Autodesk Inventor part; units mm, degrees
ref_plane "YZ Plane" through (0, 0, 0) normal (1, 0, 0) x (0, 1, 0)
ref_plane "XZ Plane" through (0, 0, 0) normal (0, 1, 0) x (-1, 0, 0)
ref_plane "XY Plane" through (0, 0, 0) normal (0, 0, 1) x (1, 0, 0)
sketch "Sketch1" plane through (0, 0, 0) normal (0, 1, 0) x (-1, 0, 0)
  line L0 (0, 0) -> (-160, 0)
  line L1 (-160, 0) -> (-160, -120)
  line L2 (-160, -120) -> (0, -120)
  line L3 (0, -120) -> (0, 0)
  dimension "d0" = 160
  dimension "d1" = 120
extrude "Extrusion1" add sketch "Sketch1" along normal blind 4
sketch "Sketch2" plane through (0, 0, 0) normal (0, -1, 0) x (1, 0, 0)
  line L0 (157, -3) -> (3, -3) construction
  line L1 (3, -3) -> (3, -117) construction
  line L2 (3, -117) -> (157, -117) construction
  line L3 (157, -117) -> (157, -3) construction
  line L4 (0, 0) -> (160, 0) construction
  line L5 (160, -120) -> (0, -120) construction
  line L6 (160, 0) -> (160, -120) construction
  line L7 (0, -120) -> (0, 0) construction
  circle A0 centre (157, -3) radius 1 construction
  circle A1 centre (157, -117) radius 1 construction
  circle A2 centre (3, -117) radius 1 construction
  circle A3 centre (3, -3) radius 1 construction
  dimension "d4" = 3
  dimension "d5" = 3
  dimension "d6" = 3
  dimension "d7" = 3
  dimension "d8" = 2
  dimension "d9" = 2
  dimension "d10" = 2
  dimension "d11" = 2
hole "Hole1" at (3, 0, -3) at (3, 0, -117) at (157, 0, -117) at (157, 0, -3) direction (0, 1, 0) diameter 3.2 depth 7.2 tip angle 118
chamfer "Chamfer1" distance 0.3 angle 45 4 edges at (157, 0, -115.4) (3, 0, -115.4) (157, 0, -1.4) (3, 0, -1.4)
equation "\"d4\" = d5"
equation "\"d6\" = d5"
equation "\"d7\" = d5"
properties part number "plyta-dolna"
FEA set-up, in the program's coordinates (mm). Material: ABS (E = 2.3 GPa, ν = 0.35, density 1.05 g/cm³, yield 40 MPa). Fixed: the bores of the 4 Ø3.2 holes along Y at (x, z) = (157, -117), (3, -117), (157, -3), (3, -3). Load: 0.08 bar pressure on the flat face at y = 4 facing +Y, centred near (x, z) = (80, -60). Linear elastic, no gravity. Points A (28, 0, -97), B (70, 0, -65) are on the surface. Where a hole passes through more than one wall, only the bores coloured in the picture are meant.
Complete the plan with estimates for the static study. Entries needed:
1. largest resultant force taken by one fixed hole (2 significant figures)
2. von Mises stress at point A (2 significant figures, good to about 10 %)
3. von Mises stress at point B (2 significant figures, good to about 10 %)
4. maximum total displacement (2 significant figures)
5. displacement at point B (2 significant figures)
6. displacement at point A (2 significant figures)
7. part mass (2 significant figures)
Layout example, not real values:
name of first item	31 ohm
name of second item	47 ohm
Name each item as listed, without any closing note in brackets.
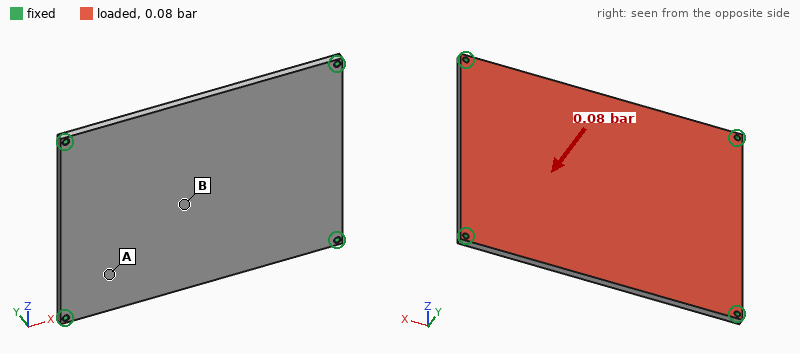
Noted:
largest resultant force taken by one fixed hole	38 N
von Mises stress at point A	1.8 MPa
von Mises stress at point B	4.0 MPa
maximum total displacement	2.3 mm
displacement at point B	2.2 mm
displacement at point A	1.0 mm
part mass	81 g
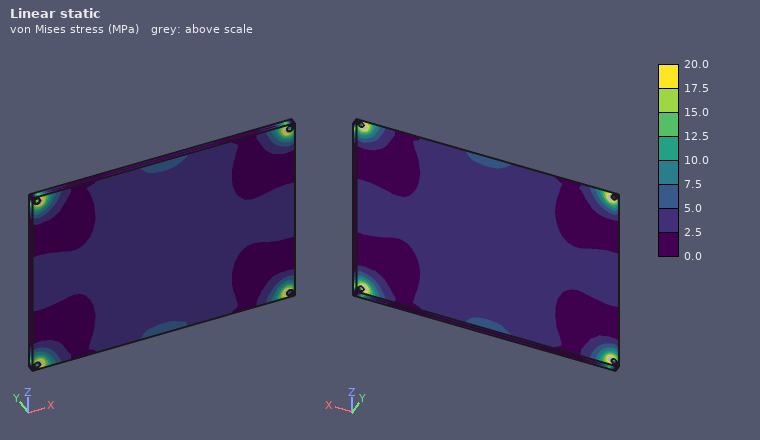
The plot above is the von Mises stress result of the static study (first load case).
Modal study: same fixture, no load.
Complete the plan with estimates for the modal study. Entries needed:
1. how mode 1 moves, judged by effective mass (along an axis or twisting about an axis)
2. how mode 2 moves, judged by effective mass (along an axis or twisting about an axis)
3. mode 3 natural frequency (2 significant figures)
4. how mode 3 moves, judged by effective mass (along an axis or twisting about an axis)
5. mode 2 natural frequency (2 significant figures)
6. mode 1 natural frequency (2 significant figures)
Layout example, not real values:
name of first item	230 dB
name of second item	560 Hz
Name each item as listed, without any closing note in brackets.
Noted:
how mode 1 moves, judged by effective mass	along Y
how mode 2 moves, judged by effective mass	twisting about X
mode 3 natural frequency	390 Hz
how mode 3 moves, judged by effective mass	twisting about Z
mode 2 natural frequency	300 Hz
mode 1 natural frequency	170 Hz
